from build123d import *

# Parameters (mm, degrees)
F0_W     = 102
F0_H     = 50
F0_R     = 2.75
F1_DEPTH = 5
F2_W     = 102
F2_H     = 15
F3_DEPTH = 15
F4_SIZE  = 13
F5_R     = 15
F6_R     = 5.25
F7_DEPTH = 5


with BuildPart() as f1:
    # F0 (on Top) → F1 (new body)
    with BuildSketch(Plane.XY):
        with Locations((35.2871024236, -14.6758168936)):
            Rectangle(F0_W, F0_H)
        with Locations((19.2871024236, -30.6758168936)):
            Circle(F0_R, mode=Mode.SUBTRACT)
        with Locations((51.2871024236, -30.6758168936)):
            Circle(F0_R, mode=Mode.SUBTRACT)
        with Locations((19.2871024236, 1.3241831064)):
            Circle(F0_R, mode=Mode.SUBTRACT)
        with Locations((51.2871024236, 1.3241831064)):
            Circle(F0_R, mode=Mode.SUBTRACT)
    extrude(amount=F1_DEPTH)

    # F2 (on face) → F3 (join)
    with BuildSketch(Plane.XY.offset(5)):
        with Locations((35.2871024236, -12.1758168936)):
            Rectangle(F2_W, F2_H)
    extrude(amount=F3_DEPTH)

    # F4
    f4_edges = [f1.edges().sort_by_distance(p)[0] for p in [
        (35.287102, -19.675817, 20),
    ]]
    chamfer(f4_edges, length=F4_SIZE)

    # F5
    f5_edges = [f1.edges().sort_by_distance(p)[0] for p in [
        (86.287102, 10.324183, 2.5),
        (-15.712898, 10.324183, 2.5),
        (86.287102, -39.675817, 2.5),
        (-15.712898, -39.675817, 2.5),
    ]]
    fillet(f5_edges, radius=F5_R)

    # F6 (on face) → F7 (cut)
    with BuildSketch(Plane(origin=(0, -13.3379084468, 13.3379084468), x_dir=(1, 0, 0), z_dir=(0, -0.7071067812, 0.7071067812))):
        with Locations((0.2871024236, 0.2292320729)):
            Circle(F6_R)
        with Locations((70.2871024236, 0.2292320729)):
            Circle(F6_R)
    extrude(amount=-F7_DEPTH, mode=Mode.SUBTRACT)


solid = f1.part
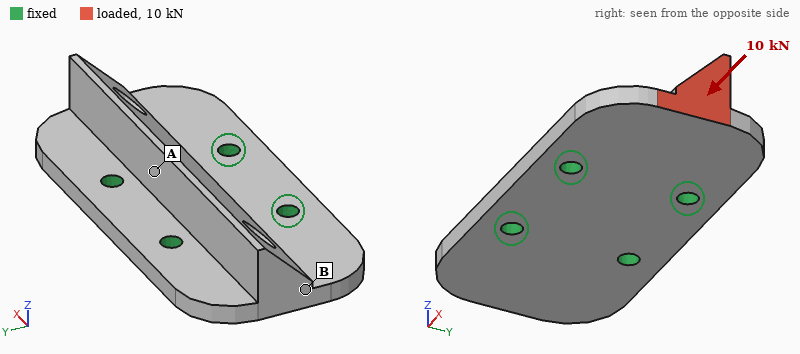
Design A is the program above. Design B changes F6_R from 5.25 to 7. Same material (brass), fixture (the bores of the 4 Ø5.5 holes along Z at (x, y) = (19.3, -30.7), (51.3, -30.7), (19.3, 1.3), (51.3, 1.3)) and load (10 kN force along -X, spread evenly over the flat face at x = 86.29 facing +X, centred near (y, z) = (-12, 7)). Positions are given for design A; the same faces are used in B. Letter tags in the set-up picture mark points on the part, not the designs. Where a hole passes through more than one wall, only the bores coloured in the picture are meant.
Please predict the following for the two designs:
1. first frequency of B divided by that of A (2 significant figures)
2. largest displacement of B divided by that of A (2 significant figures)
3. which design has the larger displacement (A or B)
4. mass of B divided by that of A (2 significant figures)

0.99
1.2
B
0.98
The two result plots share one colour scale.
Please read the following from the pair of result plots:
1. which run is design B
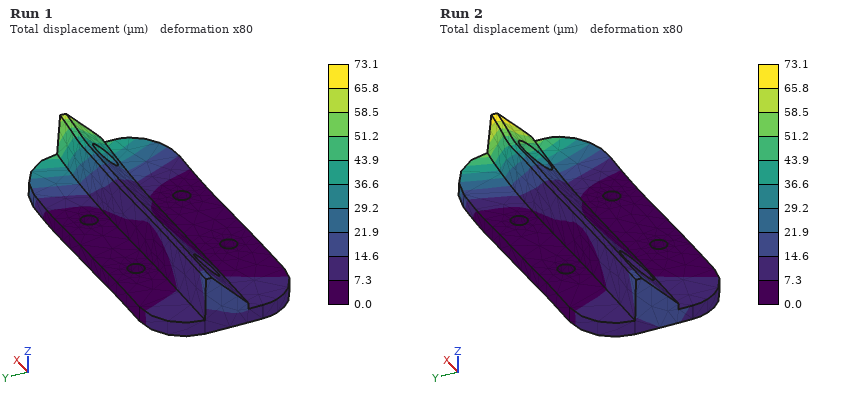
Run 2
